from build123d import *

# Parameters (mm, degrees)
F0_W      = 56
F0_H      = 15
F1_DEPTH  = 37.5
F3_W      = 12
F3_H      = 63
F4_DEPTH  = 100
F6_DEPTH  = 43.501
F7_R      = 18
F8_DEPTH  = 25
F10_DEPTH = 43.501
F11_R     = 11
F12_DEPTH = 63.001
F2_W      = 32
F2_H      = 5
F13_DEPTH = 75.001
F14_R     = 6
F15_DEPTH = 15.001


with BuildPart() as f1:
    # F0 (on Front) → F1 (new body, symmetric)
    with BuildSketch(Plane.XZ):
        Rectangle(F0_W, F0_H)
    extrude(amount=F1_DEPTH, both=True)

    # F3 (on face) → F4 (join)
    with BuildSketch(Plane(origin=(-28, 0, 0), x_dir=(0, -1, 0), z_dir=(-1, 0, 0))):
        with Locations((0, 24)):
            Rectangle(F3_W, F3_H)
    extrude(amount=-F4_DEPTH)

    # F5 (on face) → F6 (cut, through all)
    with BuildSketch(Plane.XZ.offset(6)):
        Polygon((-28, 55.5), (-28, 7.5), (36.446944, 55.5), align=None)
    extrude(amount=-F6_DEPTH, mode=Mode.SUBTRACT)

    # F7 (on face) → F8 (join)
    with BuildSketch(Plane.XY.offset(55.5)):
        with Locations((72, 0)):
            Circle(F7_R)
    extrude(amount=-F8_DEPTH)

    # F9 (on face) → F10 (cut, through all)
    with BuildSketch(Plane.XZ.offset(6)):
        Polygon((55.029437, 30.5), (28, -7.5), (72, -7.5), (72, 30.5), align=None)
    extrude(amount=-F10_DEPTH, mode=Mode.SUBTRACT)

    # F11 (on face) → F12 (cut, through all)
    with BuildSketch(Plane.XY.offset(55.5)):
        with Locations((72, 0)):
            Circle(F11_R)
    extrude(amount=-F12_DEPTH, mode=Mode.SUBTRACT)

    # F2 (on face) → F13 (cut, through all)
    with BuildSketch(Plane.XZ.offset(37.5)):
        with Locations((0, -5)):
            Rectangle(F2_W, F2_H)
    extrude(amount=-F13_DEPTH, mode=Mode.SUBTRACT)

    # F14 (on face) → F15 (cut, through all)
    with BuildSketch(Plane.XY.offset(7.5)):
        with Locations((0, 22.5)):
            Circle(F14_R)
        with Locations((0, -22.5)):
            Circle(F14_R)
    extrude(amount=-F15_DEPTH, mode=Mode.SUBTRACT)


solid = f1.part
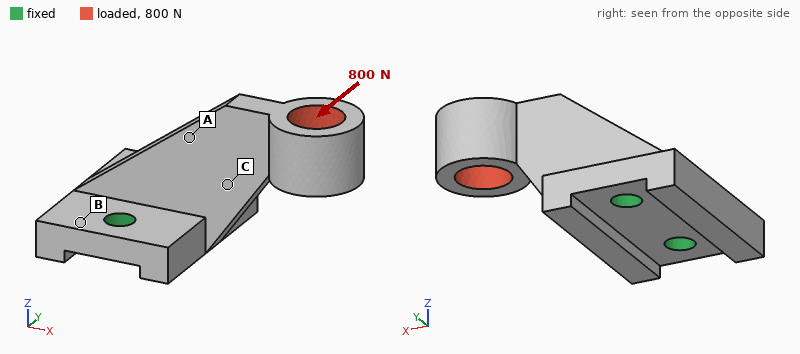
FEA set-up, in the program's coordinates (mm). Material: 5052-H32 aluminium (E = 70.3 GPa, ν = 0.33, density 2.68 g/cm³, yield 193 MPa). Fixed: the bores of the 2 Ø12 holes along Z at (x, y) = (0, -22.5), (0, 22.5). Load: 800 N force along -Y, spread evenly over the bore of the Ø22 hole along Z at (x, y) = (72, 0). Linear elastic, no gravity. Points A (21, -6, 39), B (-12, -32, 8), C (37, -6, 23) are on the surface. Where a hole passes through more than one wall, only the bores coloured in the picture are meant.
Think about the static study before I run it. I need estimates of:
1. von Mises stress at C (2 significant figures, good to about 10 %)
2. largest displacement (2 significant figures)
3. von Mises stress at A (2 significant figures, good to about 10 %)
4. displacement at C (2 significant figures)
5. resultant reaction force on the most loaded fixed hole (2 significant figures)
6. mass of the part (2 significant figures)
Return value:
40 MPa
0.37 mm
33 MPa
0.057 mm
1.5 kN
250 g
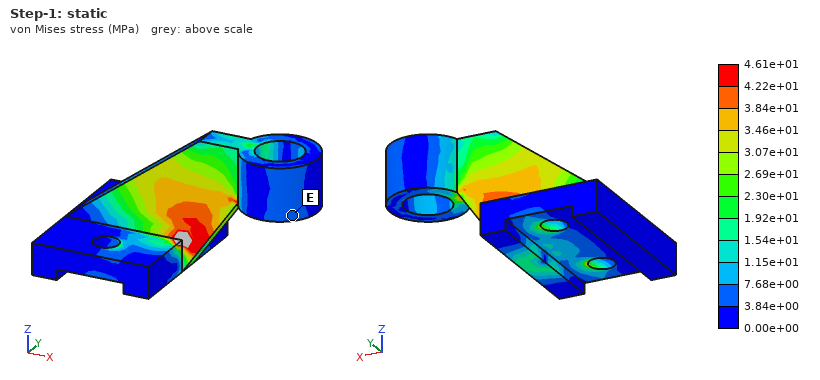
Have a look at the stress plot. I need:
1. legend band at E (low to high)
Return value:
3.84e+00 to 7.68e+00 MPa
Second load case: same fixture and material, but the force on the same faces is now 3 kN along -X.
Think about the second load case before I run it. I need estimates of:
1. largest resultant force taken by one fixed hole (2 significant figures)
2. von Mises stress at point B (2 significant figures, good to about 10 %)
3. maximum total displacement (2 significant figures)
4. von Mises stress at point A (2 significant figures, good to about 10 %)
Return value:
1.5 kN
19 MPa
0.23 mm
18 MPa
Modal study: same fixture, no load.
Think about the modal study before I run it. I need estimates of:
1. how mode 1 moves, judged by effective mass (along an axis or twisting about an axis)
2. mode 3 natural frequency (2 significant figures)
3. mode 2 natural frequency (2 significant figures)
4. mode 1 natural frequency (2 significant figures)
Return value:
along Y
3700 Hz
1800 Hz
1200 Hz
